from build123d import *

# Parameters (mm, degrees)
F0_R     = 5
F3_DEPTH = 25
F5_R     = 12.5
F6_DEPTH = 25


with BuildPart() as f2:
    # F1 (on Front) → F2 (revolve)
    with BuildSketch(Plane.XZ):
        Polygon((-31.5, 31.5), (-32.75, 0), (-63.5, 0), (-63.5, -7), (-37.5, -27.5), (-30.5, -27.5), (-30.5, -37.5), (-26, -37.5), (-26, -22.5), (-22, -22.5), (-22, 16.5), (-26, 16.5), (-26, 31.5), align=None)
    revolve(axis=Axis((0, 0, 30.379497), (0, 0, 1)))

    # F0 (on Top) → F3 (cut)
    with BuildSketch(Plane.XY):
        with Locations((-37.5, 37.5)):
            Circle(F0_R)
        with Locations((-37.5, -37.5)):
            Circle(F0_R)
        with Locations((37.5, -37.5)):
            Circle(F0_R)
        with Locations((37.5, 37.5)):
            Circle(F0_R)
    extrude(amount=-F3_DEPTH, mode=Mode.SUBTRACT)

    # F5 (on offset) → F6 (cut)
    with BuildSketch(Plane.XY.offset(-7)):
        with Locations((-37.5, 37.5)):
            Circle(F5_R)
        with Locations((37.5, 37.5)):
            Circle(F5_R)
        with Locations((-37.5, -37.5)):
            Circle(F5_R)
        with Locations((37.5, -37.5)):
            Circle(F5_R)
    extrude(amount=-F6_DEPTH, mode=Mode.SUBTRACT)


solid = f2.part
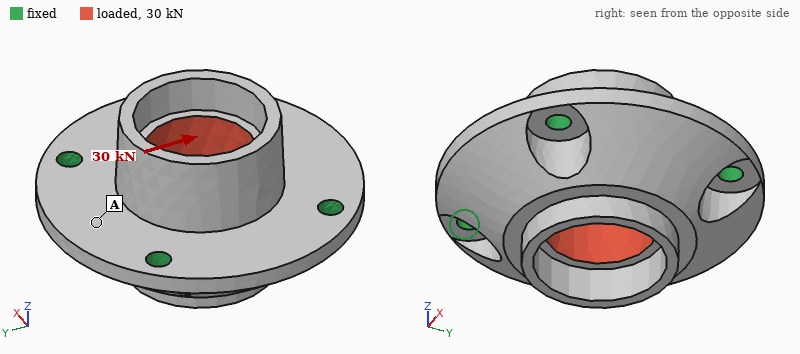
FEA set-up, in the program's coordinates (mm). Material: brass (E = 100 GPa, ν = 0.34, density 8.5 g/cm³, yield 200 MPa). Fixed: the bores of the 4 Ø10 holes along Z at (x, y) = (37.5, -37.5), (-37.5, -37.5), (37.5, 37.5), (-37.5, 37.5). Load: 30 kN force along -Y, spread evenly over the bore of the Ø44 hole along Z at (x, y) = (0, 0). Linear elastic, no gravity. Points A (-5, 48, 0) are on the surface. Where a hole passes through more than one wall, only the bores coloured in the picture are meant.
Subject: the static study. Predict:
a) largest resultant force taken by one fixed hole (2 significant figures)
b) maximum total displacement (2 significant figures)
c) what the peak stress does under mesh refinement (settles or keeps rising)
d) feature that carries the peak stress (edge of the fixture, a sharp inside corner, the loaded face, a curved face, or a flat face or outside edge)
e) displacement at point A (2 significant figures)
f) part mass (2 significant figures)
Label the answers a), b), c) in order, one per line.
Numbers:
a) 7.5 kN
b) 15 µm
c) keeps rising
d) edge of the fixture
e) 8.9 µm
f) 2.1 kg
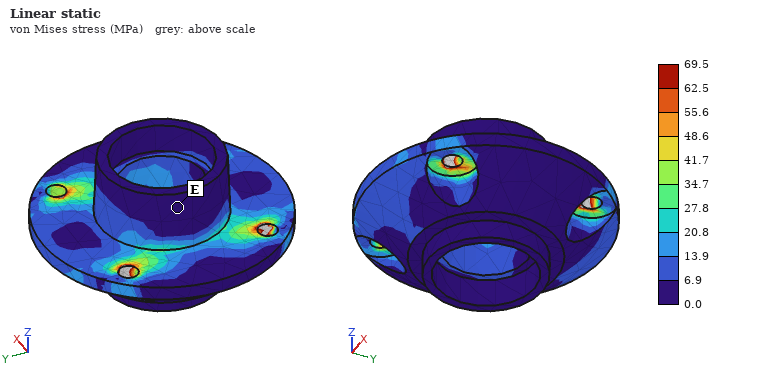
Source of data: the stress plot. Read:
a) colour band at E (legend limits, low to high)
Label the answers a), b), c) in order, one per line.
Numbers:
a) 0.0 to 6.9 MPa
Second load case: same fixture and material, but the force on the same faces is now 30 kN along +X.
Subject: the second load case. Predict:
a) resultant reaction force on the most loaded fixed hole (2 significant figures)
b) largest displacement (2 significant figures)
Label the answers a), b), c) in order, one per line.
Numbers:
a) 7.5 kN
b) 15 µm
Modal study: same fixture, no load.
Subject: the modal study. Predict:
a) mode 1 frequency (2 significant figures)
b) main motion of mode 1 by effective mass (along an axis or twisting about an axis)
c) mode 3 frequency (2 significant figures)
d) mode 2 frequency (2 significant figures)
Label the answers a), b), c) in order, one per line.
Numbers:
a) 4500 Hz
b) along Z
c) 5000 Hz
d) 5000 Hz
